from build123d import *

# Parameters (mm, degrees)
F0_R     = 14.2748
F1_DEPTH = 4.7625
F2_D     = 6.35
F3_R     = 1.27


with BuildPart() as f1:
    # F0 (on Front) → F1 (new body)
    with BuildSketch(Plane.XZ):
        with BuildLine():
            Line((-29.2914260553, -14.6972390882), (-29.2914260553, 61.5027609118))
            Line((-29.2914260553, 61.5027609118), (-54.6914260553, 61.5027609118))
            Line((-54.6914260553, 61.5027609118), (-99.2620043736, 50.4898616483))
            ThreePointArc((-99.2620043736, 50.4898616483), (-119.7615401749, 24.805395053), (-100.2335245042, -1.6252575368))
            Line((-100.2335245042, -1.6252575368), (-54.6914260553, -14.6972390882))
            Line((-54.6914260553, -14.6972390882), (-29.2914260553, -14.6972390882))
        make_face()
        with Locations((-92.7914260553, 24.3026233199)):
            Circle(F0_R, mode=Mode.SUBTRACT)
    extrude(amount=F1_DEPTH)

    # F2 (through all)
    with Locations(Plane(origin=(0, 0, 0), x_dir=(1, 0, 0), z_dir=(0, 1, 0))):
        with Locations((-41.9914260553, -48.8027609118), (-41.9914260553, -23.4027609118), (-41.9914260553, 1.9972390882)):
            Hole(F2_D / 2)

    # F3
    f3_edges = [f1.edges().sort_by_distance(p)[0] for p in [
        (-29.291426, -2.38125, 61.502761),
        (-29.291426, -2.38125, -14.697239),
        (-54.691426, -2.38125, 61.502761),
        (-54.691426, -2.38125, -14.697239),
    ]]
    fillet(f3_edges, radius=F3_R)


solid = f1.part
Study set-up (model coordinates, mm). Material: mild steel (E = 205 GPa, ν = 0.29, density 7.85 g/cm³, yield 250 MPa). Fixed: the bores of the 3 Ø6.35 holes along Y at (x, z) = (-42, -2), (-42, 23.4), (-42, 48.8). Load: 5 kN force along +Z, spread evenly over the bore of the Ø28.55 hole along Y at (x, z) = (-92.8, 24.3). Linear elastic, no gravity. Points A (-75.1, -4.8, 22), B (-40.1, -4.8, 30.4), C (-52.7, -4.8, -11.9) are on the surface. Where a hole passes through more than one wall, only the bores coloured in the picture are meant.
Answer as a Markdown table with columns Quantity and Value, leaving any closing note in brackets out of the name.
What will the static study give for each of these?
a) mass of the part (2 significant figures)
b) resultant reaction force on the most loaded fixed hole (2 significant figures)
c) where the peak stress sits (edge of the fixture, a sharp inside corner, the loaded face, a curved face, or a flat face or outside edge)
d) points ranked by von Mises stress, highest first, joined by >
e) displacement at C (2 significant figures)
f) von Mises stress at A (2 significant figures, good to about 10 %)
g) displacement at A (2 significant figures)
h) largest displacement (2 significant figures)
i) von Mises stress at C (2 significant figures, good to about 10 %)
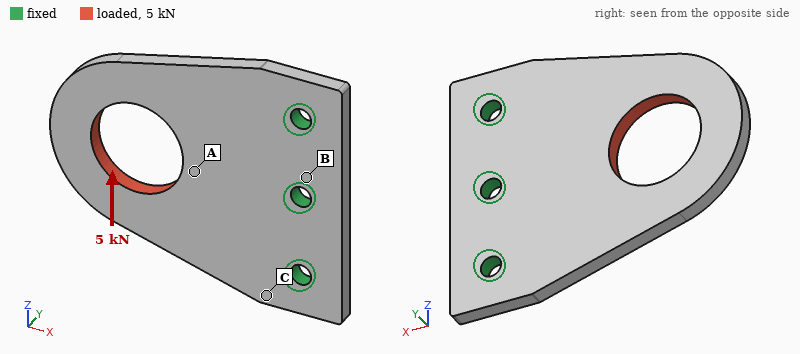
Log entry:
| Quantity | Value |
|---|---|
| mass of the part | 180 g |
| resultant reaction force on the most loaded fixed hole | 4.9 kN |
| where the peak stress sits | edge of the fixture |
| points ranked by von Mises stress, highest first, joined by > | A > C > B |
| displacement at C | 5.9 µm |
| von Mises stress at A | 55 MPa |
| displacement at A | 11 µm |
| largest displacement | 39 µm |
| von Mises stress at C | 32 MPa |
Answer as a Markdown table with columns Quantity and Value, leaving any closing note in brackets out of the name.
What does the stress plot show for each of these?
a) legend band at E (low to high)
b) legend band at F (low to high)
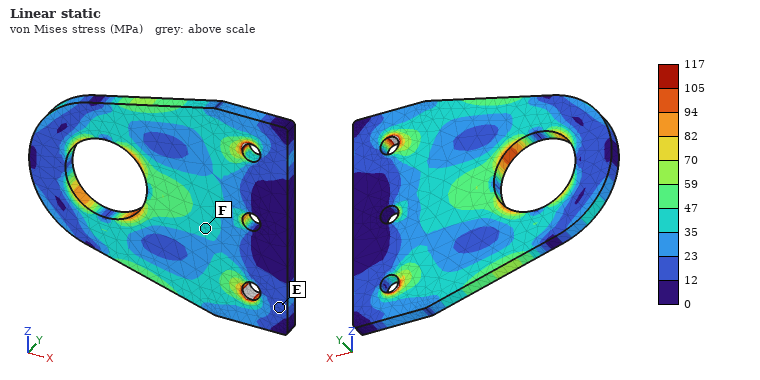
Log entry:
| Quantity | Value |
|---|---|
| legend band at E | 12 to 23 MPa |
| legend band at F | 35 to 47 MPa |
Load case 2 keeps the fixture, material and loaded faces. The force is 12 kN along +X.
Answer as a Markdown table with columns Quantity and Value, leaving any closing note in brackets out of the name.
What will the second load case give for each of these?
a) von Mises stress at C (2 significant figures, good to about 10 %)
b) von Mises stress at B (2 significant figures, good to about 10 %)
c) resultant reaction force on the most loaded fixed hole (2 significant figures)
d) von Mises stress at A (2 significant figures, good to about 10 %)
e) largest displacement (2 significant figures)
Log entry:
| Quantity | Value |
|---|---|
| von Mises stress at C | 21 MPa |
| von Mises stress at B | 16 MPa |
| resultant reaction force on the most loaded fixed hole | 4.5 kN |
| von Mises stress at A | 37 MPa |
| largest displacement | 23 µm |
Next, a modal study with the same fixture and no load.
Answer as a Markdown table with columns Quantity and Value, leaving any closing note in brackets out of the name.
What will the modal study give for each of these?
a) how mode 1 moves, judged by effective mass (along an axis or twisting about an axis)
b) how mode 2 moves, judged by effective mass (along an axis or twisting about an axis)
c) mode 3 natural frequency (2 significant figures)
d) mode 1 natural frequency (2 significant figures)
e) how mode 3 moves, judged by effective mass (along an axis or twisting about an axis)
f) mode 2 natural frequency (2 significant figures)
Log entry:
| Quantity | Value |
|---|---|
| how mode 1 moves, judged by effective mass | along Y |
| how mode 2 moves, judged by effective mass | twisting about X |
| mode 3 natural frequency | 4100 Hz |
| mode 1 natural frequency | 960 Hz |
| how mode 3 moves, judged by effective mass | along Y |
| mode 2 natural frequency | 2600 Hz |
